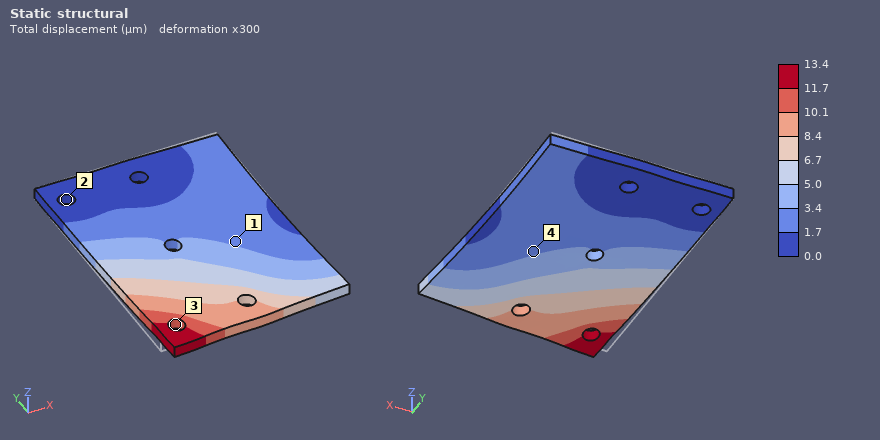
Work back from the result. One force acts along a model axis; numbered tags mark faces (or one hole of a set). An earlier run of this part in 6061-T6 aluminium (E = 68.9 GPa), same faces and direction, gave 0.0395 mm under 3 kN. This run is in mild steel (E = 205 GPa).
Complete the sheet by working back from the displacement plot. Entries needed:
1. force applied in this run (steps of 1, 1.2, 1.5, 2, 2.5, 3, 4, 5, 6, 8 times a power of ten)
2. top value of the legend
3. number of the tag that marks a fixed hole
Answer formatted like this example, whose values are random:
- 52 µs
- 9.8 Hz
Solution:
- 3 kN
- 13.4 µm
- 2
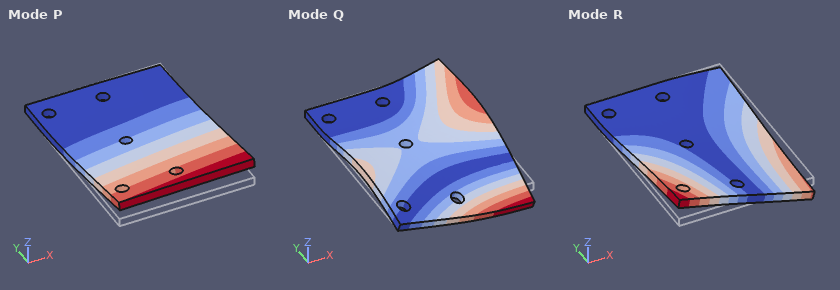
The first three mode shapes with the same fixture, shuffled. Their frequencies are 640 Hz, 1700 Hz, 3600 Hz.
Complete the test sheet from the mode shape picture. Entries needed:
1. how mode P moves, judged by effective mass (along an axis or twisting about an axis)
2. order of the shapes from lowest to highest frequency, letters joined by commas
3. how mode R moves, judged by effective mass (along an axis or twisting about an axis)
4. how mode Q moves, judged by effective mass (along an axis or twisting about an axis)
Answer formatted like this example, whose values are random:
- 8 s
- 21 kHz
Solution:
- along Z
- P, R, Q
- twisting about Y
- along Z
